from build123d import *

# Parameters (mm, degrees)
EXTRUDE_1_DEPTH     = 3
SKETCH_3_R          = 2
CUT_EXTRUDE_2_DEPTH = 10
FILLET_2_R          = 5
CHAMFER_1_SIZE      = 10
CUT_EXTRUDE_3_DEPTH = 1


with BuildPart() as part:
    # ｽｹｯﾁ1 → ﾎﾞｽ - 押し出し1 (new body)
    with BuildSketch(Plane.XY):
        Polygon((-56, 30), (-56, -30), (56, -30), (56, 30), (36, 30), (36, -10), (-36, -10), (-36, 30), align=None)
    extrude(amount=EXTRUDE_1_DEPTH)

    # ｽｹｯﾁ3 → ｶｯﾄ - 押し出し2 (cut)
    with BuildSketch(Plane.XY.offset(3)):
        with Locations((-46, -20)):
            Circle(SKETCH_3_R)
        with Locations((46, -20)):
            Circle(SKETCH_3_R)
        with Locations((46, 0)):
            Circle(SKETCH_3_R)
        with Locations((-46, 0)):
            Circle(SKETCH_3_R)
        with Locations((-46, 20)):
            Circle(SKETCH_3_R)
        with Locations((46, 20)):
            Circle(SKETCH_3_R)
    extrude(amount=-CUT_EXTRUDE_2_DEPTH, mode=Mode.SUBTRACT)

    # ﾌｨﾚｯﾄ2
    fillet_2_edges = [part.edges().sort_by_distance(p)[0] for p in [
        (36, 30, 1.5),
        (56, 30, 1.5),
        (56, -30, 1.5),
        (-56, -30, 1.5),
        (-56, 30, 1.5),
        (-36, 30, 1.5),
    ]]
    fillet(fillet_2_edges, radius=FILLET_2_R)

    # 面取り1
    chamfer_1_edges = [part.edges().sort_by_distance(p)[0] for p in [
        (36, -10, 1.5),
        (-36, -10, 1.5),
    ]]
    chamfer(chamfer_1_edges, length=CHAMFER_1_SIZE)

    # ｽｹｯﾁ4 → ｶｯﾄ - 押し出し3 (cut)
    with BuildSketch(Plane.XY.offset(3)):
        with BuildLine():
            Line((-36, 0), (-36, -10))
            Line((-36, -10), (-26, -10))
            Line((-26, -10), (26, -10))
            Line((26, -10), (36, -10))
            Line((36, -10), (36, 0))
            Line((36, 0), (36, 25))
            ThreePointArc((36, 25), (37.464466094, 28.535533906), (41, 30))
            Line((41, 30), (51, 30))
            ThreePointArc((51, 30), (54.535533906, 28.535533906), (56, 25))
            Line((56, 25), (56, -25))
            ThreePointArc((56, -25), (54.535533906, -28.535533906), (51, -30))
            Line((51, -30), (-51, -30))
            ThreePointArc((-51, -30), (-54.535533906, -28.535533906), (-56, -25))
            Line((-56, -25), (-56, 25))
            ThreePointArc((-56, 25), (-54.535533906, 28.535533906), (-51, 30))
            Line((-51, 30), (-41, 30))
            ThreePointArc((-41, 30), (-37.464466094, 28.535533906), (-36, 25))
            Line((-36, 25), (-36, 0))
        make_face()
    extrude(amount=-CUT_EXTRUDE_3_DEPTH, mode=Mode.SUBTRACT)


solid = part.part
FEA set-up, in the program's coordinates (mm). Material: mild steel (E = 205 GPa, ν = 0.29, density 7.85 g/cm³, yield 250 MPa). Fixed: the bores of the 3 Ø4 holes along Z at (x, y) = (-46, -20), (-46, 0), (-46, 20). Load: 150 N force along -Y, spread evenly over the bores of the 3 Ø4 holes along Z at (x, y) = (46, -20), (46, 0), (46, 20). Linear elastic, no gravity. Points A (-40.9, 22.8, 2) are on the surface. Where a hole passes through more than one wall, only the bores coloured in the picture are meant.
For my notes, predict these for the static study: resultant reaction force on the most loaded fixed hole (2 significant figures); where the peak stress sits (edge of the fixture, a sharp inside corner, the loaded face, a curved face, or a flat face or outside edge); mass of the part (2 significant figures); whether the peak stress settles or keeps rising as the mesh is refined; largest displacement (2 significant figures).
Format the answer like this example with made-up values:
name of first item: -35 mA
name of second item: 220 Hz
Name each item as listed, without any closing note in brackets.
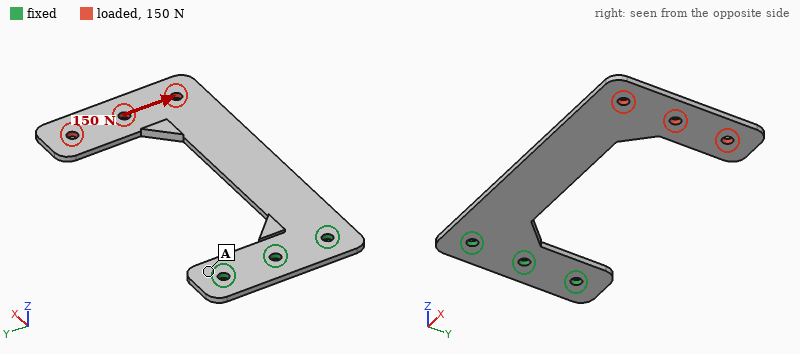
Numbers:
resultant reaction force on the most loaded fixed hole: 590 N
where the peak stress sits: a sharp inside corner
mass of the part: 61 g
whether the peak stress settles or keeps rising as the mesh is refined: keeps rising
largest displacement: 0.16 mm
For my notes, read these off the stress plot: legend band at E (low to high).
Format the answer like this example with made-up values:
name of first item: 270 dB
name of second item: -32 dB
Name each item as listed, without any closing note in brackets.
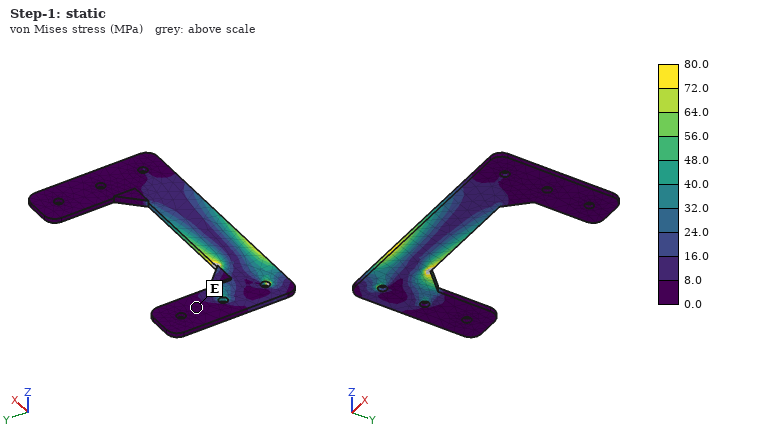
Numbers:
legend band at E: 0.0 to 8.0 MPa
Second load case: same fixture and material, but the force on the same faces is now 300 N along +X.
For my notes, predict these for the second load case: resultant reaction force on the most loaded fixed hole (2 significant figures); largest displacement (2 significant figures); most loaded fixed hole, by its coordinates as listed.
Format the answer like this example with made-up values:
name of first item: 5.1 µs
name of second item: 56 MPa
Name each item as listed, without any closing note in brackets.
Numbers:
resultant reaction force on the most loaded fixed hole: 270 N
largest displacement: 0.13 mm
most loaded fixed hole, by its coordinates as listed: (-46, 0)
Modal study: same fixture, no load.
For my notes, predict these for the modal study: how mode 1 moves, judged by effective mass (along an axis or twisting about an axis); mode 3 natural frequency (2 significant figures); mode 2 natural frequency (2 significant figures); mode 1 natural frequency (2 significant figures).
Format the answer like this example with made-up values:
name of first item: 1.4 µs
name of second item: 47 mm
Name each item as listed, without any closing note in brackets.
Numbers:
how mode 1 moves, judged by effective mass: along Z
mode 3 natural frequency: 1000 Hz
mode 2 natural frequency: 430 Hz
mode 1 natural frequency: 120 Hz
